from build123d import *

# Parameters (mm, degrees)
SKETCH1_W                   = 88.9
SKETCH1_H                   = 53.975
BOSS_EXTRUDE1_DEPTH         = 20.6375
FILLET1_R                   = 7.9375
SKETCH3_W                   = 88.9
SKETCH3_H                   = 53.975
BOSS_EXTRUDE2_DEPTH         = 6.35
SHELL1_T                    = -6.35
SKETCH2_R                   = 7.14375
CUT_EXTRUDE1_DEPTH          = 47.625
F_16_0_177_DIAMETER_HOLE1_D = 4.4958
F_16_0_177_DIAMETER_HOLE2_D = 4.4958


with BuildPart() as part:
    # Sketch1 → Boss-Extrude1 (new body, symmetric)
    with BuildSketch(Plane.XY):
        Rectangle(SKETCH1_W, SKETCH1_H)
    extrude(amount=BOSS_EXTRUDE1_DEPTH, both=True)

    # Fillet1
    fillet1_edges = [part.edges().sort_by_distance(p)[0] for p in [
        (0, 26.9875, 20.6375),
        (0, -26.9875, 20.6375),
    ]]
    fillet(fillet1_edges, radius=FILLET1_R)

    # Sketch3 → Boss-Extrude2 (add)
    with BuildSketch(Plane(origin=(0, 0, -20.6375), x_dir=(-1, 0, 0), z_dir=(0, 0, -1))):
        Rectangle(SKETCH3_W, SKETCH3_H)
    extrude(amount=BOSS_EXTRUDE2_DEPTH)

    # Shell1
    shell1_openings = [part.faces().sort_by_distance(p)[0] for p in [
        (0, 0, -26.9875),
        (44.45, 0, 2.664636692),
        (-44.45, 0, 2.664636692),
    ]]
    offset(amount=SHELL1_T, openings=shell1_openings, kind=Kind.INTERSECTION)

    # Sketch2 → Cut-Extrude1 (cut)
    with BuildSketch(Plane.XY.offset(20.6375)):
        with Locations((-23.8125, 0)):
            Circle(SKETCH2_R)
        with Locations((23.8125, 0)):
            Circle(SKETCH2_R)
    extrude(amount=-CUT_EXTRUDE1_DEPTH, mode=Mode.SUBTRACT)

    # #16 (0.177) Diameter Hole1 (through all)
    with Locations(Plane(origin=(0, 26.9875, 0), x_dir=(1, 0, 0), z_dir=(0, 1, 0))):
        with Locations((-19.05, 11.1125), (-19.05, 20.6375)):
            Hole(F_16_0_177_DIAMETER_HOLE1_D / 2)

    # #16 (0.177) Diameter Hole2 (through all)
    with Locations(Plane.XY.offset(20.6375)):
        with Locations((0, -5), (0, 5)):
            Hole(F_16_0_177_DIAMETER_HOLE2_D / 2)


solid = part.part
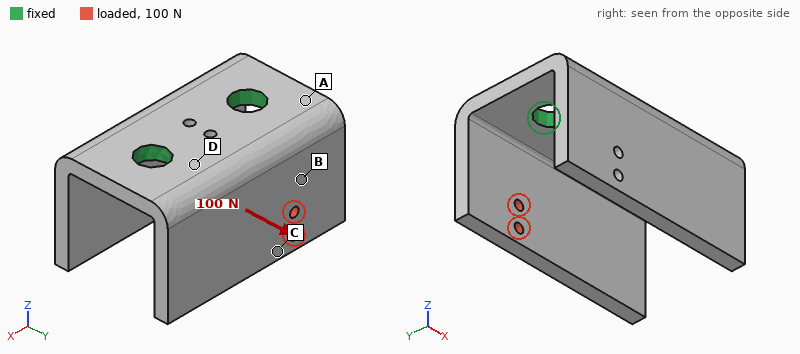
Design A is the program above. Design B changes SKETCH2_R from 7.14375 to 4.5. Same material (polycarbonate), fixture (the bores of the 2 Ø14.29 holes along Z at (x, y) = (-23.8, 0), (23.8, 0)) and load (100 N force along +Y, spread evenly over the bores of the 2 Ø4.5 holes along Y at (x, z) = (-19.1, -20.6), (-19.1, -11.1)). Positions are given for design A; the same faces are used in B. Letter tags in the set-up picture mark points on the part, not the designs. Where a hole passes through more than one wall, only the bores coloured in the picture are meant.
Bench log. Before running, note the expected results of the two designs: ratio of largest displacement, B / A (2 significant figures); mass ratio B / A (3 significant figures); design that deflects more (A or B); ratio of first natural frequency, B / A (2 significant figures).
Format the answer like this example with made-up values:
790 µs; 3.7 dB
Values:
1.1; 1.02; B; 0.90
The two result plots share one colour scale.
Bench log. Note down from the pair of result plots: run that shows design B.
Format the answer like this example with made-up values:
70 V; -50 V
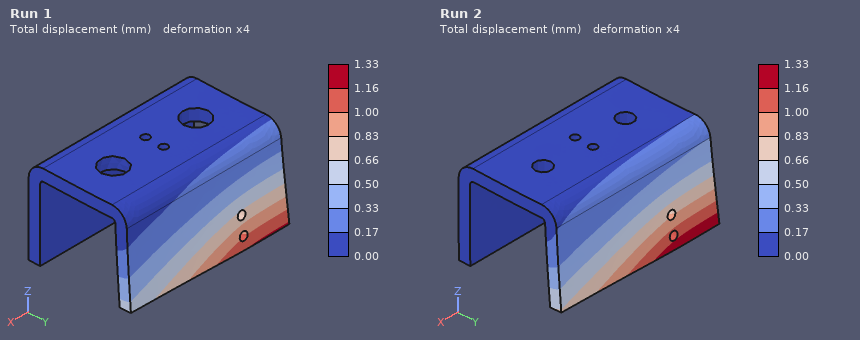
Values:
Run 2
